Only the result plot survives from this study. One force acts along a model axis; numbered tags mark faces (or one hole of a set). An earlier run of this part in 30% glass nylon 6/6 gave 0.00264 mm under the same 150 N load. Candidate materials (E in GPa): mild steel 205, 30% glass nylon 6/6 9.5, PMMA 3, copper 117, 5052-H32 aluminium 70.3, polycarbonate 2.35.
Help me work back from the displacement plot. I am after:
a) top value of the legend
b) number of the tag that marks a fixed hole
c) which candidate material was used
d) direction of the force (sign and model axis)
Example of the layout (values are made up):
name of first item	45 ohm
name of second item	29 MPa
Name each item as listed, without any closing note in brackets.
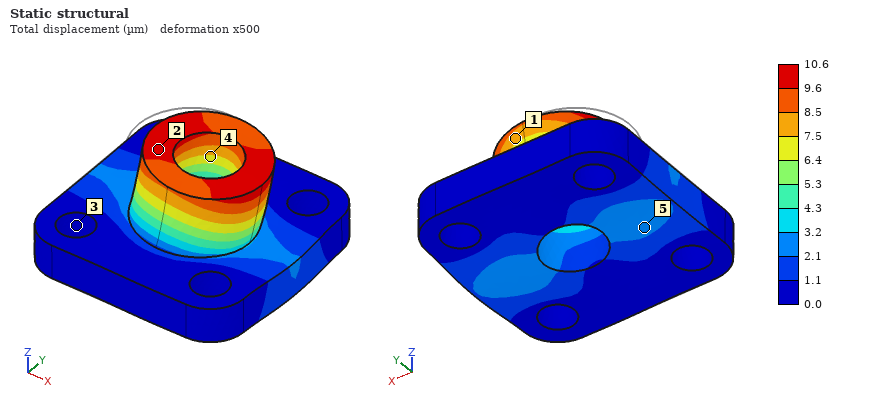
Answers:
top value of the legend	10.6 µm
number of the tag that marks a fixed hole	3
which candidate material was used	polycarbonate
direction of the force	+X
